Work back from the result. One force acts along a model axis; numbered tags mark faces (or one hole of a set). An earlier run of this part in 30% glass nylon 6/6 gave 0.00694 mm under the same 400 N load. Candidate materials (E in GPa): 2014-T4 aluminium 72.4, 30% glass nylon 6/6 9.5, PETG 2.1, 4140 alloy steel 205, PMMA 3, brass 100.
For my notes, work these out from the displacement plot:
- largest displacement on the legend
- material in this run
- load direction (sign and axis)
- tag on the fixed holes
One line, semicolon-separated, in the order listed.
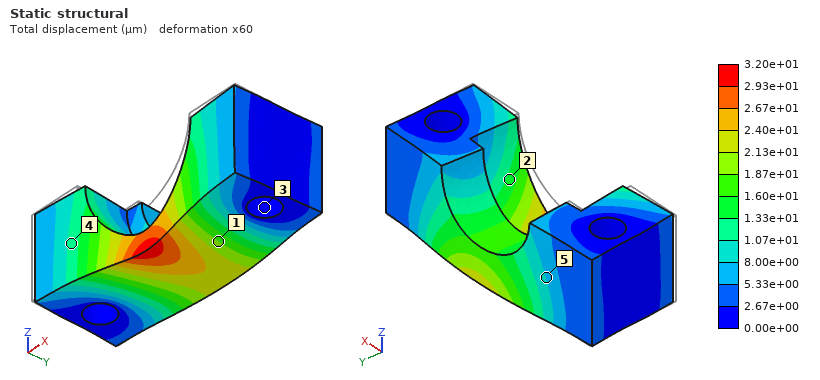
3.20e+01 µm; PETG; +Y; 3
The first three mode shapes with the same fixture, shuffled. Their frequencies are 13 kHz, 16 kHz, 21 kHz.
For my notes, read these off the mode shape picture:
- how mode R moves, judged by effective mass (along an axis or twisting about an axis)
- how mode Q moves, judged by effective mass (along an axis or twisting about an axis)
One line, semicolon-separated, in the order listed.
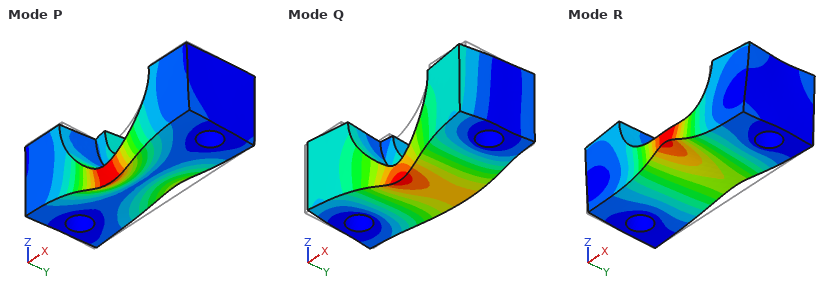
along Z; along Y
